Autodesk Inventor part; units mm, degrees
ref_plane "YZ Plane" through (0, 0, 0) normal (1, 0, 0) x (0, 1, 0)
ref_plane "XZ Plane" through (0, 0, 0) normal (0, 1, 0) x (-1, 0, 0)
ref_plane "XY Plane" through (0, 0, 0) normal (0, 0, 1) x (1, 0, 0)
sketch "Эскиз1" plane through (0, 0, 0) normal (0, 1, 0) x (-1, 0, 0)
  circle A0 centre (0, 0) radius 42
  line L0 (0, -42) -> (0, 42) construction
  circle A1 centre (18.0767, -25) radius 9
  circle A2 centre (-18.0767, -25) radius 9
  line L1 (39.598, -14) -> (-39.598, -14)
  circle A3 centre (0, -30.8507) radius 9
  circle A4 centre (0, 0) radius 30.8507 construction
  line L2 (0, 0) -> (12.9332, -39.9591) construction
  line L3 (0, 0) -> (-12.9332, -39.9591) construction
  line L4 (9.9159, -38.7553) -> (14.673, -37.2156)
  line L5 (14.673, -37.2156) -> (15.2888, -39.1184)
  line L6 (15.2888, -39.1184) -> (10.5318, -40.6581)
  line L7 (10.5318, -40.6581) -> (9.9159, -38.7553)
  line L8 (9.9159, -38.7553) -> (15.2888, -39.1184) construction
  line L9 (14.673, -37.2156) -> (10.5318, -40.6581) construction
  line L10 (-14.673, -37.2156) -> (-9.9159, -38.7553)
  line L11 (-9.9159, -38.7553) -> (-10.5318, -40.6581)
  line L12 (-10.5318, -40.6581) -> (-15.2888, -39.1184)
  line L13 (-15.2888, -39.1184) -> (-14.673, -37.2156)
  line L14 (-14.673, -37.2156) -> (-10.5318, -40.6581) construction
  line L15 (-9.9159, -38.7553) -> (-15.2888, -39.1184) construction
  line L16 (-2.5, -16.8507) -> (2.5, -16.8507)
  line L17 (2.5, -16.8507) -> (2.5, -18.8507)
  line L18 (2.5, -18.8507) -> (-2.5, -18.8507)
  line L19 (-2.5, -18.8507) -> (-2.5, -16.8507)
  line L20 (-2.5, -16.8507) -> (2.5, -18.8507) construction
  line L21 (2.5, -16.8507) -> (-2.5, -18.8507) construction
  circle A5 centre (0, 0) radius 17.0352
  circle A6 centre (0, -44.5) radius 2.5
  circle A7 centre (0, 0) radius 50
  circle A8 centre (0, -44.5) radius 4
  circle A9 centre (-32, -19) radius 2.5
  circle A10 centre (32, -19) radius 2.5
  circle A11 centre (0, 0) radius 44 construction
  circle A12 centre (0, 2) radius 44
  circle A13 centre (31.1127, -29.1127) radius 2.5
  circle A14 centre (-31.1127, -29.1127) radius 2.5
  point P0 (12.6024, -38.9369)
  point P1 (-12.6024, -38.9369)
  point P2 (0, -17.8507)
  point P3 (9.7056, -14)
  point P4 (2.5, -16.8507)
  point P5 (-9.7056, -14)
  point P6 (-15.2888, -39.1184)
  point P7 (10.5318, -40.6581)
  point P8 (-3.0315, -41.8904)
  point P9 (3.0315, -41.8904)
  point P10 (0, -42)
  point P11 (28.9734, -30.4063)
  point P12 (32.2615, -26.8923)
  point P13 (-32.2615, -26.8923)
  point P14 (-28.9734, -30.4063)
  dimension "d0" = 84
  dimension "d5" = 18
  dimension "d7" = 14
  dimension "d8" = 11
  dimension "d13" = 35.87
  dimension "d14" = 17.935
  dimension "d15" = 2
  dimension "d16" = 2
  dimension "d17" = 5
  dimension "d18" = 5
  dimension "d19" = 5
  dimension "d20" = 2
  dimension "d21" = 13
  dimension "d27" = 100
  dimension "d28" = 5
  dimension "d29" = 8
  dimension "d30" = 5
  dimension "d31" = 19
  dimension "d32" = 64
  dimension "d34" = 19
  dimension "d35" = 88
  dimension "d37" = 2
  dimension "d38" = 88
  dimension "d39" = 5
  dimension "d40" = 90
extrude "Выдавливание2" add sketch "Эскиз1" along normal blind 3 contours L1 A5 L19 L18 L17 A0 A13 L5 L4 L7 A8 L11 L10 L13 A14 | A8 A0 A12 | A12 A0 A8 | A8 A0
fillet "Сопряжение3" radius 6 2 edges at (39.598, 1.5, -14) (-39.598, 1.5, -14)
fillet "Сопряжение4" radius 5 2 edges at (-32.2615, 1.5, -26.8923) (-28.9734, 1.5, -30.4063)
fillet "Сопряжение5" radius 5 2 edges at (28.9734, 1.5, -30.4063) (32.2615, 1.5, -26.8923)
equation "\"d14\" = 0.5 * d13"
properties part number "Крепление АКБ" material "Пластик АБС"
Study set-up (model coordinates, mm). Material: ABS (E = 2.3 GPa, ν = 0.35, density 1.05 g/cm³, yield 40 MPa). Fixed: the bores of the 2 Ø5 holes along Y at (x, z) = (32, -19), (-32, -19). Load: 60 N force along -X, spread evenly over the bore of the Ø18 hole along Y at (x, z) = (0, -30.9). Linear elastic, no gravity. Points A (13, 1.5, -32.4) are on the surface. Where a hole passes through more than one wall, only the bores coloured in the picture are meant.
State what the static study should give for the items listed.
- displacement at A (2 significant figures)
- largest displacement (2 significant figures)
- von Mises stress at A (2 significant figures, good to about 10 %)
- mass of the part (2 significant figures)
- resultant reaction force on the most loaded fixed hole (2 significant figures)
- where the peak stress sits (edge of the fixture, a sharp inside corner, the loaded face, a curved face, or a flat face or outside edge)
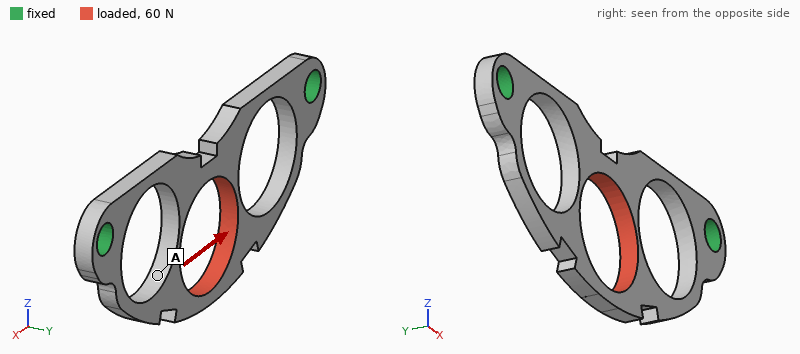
0.11 mm
0.12 mm
1.8 MPa
2.1 g
32 N
a curved face
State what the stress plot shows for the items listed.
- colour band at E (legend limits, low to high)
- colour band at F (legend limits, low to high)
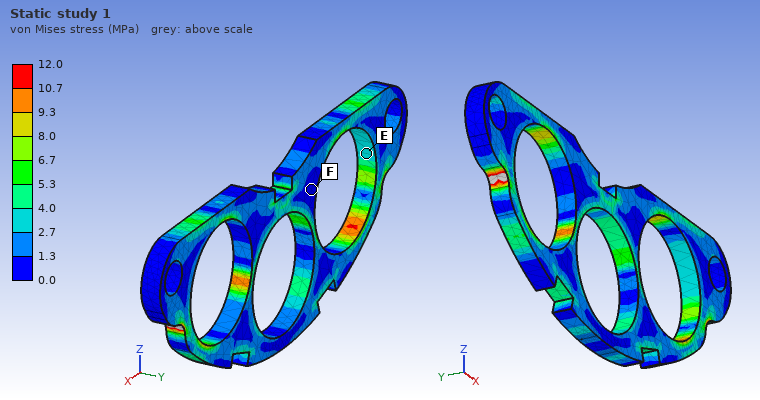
2.7 to 4.0 MPa
0.0 to 1.3 MPa
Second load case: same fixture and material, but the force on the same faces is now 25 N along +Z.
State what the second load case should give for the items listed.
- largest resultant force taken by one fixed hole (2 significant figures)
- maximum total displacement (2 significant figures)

19 N
0.14 mm
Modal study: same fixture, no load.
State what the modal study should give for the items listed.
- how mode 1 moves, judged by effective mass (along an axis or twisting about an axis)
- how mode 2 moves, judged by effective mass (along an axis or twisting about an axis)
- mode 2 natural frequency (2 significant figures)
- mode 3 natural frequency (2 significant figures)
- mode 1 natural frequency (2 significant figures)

along Y
along Y
1300 Hz
1900 Hz
640 Hz
